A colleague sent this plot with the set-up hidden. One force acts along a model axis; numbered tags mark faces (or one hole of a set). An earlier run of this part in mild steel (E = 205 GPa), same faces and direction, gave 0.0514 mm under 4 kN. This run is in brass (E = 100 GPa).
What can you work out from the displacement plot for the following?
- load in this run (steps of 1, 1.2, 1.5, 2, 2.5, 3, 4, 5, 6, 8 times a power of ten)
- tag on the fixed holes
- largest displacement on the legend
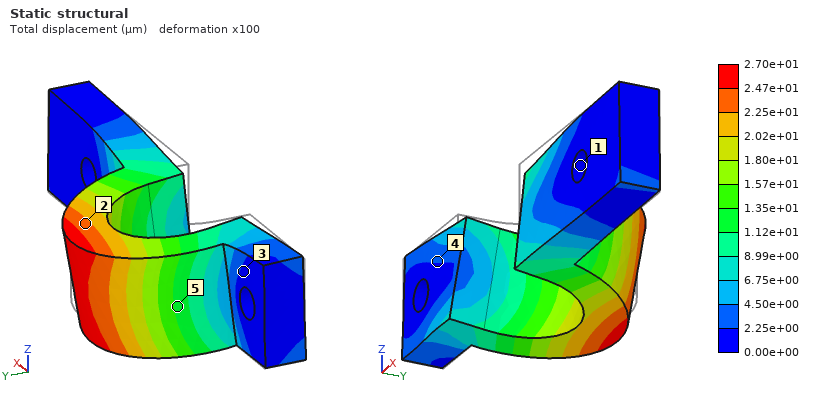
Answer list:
1 kN
1
2.70e+01 µm
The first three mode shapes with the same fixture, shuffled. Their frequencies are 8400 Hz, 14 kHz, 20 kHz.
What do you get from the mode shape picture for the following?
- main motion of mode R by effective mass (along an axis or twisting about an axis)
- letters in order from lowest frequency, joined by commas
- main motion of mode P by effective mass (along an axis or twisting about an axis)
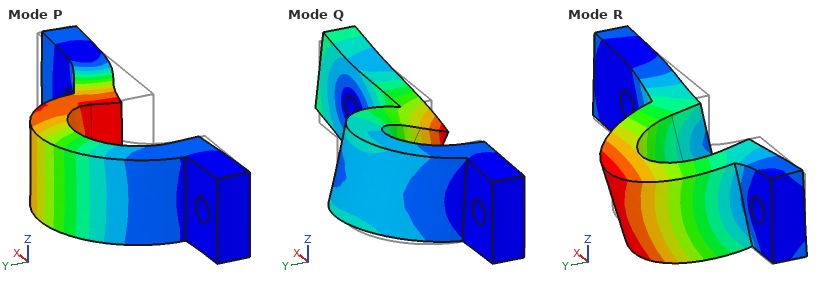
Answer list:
along Z
R, P, Q
along Y
